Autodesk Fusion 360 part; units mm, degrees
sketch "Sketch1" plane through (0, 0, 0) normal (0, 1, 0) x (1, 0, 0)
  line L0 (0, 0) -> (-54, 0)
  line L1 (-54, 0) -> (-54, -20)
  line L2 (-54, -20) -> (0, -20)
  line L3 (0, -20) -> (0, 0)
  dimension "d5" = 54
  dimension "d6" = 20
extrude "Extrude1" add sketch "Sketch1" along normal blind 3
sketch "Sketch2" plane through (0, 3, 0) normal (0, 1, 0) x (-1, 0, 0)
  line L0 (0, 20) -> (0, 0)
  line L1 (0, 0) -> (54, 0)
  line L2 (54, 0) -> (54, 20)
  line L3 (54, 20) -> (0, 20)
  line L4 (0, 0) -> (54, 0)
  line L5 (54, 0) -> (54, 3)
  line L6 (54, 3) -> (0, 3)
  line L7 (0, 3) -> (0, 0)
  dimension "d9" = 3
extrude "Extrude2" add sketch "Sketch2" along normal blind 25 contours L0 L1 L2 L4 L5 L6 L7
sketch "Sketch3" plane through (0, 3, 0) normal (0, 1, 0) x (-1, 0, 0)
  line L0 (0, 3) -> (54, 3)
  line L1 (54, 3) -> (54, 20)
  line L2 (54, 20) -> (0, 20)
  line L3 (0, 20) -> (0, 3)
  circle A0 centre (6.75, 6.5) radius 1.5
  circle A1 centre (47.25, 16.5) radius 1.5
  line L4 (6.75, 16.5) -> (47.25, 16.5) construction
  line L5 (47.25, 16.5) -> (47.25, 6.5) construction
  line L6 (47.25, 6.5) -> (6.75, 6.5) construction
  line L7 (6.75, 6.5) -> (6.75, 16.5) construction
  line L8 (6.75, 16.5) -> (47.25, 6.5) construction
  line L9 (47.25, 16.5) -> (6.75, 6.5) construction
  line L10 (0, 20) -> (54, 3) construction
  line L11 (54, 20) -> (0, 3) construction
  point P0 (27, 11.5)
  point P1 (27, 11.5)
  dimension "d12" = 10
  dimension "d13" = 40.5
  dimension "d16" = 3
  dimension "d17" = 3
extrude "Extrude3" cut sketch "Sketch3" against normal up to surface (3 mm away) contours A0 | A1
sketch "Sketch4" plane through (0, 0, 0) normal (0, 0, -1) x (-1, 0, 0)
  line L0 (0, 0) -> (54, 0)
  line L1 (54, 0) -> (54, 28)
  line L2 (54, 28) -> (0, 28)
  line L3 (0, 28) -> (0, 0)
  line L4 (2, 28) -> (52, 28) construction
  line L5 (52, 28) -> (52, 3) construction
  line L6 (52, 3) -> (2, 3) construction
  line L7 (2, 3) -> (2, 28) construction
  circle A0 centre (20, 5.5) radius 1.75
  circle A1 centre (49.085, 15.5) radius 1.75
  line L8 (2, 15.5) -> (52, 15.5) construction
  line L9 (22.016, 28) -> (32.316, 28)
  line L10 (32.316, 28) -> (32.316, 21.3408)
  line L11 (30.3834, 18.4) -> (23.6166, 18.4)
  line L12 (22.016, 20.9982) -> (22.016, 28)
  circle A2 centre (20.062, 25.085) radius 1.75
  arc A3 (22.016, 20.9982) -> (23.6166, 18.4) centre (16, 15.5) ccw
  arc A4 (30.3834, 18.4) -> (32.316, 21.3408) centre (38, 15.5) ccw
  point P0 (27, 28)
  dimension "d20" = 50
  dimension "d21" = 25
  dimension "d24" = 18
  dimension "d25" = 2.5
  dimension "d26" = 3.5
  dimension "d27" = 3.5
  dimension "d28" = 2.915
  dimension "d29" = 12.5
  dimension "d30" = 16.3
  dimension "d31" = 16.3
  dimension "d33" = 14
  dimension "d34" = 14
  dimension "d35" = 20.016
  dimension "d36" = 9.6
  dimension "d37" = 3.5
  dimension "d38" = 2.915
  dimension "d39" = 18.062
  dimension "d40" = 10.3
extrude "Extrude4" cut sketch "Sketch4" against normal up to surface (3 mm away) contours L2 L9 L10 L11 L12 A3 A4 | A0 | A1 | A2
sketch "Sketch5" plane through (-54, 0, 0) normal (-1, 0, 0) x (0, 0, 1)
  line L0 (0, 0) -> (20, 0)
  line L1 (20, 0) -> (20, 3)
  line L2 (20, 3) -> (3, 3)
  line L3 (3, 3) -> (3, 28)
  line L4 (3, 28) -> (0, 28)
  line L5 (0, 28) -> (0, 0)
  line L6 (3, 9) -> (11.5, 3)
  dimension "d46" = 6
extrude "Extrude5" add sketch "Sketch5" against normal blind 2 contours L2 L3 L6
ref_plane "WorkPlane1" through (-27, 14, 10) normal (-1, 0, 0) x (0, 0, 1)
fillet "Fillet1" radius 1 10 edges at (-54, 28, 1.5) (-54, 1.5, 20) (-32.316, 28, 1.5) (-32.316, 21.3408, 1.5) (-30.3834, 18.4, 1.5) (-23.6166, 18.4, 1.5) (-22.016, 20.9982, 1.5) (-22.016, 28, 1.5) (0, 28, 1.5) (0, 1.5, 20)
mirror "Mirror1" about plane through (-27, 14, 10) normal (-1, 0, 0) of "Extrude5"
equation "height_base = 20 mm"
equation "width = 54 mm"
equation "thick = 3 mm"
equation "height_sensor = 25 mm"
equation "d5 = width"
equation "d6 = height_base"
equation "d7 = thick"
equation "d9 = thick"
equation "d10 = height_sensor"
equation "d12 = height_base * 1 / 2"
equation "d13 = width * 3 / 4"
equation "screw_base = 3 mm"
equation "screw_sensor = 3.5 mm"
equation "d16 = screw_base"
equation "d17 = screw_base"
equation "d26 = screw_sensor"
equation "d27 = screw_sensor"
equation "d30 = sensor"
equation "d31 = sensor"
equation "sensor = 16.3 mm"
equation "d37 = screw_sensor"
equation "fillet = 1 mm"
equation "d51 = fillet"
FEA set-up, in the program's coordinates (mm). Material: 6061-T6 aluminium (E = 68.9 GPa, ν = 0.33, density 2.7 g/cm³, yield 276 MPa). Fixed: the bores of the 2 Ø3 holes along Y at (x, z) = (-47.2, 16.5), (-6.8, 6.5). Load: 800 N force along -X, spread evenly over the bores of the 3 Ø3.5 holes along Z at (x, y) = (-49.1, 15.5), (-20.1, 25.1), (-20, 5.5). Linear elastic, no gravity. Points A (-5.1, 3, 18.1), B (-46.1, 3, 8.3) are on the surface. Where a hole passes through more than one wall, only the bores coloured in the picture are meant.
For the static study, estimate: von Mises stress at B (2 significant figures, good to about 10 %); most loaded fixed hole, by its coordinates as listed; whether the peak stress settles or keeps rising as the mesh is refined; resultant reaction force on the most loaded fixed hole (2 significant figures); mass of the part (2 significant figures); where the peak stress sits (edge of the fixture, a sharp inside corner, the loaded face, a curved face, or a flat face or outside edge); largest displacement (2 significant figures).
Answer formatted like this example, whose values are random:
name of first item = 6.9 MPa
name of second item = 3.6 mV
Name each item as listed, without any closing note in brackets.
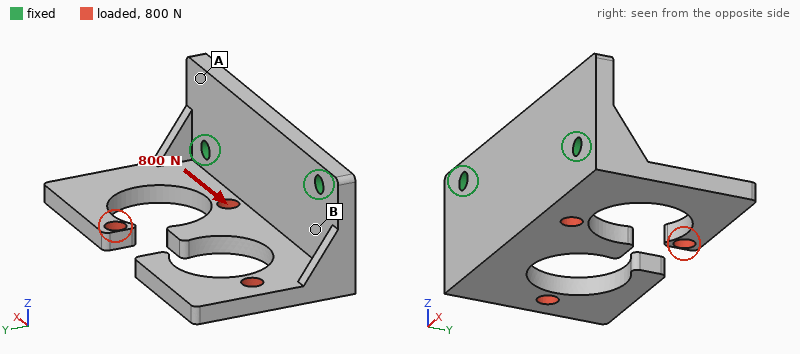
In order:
von Mises stress at B = 40 MPa
most loaded fixed hole, by its coordinates as listed = (-6.8, 6.5)
whether the peak stress settles or keeps rising as the mesh is refined = keeps rising
resultant reaction force on the most loaded fixed hole = 550 N
mass of the part = 15 g
where the peak stress sits = edge of the fixture
largest displacement = 0.20 mm
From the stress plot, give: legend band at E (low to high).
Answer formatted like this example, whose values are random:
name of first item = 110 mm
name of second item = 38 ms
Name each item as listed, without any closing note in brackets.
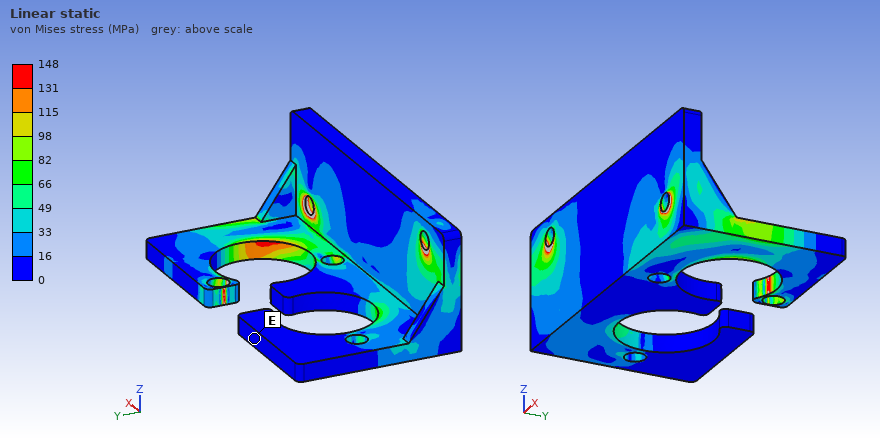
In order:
legend band at E = 0 to 16 MPa
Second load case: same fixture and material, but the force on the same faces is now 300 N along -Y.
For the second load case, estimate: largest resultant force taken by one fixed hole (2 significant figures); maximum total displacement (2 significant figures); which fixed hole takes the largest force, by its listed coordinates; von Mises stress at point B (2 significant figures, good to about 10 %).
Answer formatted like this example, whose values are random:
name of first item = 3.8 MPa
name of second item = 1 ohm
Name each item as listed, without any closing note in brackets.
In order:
largest resultant force taken by one fixed hole = 170 N
maximum total displacement = 0.14 mm
which fixed hole takes the largest force, by its listed coordinates = (-6.8, 6.5)
von Mises stress at point B = 22 MPa
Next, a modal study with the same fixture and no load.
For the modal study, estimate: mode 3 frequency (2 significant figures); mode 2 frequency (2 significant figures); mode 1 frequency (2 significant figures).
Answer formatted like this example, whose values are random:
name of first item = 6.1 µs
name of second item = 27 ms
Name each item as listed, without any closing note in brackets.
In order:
mode 3 frequency = 4600 Hz
mode 2 frequency = 2800 Hz
mode 1 frequency = 2100 Hz
